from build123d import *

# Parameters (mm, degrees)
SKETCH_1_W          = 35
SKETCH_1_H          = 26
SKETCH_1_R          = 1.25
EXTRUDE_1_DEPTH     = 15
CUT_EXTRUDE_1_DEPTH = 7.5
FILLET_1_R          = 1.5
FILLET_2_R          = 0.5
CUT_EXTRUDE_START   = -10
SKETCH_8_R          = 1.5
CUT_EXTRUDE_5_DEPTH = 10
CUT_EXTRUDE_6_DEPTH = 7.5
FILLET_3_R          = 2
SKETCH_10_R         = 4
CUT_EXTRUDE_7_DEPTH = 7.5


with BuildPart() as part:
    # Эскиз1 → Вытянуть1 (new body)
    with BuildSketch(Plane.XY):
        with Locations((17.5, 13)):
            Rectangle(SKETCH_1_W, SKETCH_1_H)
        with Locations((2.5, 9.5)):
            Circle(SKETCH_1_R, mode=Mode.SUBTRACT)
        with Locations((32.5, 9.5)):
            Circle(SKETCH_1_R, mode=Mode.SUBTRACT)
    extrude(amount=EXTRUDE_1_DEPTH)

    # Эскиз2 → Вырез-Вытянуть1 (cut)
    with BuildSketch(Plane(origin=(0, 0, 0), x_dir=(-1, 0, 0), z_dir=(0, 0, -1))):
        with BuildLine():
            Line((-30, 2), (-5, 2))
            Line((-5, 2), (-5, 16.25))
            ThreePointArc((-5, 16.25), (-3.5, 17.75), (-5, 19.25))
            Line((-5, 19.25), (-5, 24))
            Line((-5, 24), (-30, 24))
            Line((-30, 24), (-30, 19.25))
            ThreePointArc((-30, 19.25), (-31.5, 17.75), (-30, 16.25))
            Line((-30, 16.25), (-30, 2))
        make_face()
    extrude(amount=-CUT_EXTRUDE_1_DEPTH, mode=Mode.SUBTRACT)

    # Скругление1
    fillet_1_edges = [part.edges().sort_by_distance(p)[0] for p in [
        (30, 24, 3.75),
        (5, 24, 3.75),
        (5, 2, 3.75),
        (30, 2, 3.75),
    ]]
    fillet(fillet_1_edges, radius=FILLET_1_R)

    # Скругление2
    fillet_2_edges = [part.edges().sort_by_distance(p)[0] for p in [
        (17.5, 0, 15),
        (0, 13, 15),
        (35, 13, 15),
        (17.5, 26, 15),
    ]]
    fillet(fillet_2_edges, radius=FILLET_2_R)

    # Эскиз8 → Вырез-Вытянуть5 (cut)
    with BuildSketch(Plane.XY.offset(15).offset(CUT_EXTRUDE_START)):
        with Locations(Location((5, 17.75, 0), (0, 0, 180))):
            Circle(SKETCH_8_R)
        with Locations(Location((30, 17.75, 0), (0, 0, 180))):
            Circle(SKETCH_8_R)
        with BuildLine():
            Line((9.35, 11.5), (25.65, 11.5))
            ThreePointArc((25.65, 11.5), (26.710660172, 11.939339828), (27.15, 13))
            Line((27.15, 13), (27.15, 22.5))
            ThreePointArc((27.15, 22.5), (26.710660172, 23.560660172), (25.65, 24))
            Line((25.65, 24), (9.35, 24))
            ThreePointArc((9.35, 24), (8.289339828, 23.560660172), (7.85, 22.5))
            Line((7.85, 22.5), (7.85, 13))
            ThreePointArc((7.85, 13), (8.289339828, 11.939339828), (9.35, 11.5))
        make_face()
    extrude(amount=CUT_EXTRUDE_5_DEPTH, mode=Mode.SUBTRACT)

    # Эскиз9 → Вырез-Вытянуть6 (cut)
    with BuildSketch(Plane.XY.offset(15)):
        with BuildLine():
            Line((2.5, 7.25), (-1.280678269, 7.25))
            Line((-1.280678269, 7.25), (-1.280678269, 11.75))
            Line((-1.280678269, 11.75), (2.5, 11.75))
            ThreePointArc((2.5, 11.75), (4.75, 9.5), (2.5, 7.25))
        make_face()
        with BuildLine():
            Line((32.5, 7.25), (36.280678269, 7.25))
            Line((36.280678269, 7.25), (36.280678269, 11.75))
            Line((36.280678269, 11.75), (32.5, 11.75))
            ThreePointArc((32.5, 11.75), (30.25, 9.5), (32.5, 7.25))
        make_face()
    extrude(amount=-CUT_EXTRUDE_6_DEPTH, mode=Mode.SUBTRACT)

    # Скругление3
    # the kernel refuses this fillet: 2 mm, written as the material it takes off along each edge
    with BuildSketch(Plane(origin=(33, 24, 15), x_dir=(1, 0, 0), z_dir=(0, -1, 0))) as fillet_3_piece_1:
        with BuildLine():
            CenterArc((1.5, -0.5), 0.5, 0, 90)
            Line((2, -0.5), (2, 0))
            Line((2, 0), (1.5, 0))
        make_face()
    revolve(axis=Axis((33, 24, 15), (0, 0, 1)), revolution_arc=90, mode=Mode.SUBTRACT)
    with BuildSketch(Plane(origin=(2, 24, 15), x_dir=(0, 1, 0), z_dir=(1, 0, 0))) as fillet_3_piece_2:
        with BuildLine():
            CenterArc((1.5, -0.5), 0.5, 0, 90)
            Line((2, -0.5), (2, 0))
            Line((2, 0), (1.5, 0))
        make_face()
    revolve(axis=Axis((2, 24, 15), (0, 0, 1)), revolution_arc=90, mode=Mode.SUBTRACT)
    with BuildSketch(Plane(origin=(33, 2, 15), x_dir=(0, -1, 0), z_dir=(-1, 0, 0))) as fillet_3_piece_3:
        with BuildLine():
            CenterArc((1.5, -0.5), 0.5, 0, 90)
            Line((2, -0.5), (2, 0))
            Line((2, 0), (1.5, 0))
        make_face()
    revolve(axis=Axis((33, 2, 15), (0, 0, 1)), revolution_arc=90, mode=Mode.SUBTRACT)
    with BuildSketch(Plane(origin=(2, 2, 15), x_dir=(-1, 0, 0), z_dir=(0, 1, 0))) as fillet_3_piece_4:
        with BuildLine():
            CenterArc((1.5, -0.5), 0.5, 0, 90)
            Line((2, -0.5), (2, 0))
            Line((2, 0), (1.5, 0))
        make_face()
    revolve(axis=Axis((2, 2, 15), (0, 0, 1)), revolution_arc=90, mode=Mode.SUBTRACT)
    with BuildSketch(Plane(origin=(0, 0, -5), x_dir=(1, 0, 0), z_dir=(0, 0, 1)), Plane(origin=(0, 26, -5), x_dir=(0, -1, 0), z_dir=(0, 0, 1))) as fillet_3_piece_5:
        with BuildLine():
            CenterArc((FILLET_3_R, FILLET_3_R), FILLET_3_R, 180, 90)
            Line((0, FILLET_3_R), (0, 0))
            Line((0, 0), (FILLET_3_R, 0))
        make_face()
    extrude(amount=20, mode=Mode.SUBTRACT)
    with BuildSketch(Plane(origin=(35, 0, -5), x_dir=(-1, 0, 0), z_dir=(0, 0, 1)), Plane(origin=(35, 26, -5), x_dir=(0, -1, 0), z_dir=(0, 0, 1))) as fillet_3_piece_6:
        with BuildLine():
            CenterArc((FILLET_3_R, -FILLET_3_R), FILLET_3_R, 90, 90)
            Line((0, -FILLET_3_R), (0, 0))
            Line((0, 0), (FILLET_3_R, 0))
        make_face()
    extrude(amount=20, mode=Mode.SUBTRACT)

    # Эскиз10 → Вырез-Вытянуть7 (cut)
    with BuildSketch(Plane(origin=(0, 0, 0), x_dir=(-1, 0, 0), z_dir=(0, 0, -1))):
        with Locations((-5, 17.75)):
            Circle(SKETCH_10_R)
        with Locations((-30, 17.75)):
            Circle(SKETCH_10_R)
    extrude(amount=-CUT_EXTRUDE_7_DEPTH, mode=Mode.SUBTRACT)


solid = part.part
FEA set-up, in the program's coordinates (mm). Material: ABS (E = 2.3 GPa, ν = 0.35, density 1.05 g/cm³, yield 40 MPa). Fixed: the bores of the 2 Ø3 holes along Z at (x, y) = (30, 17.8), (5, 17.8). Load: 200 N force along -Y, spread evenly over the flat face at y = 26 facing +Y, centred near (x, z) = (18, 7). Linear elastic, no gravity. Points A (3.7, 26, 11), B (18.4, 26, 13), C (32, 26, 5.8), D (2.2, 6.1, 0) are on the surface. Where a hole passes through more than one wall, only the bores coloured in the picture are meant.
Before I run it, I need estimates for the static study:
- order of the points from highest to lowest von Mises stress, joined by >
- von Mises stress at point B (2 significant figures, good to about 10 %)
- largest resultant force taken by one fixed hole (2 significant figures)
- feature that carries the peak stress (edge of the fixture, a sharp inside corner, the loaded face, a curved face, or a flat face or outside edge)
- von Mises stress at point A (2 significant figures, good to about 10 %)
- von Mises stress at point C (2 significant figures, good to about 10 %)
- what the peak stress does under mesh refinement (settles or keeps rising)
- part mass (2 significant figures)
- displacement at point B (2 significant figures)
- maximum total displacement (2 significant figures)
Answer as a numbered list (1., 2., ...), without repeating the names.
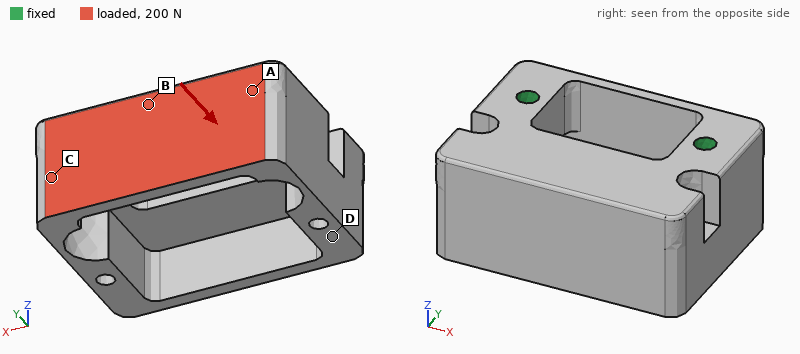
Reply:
1. B > C > A > D
2. 12 MPa
3. 110 N
4. a sharp inside corner
5. 3.0 MPa
6. 5.7 MPa
7. keeps rising
8. 7.2 g
9. 0.13 mm
10. 0.37 mm
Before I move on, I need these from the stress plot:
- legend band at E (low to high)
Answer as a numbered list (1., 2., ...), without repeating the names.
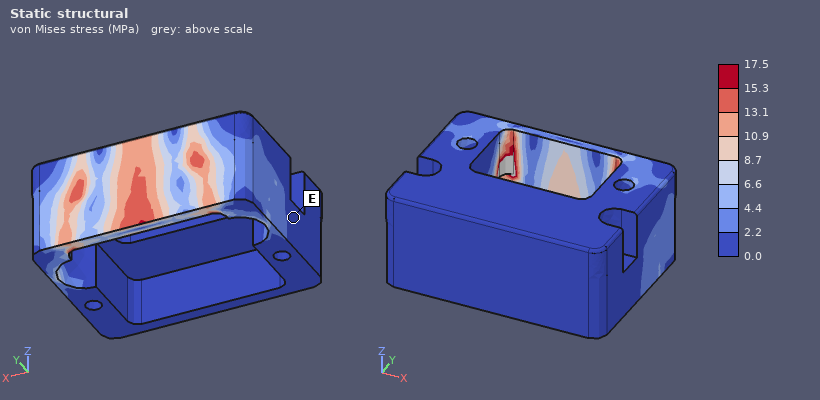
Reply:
1. 0.0 to 2.2 MPa
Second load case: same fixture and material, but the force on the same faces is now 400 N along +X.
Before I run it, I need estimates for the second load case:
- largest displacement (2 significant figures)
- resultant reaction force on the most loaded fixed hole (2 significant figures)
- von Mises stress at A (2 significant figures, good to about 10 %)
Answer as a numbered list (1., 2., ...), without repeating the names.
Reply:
1. 0.14 mm
2. 210 N
3. 3.0 MPa
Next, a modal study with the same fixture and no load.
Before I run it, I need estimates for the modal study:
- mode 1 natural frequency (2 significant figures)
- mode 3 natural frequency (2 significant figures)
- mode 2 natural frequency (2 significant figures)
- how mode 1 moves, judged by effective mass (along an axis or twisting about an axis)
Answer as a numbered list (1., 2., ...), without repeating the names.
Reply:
1. 3000 Hz
2. 5100 Hz
3. 4100 Hz
4. along Z
